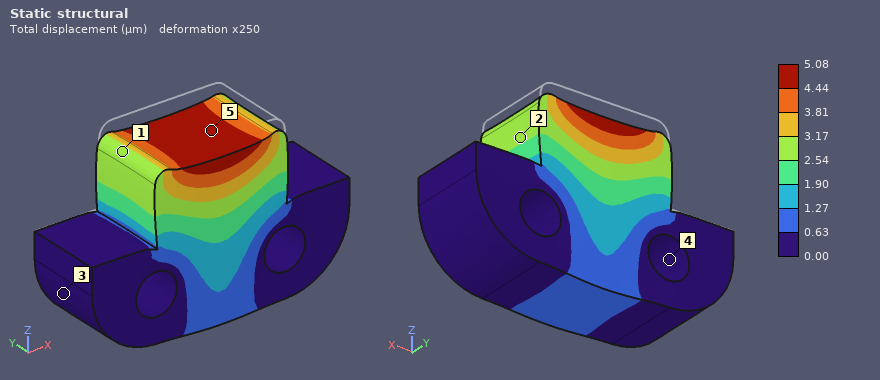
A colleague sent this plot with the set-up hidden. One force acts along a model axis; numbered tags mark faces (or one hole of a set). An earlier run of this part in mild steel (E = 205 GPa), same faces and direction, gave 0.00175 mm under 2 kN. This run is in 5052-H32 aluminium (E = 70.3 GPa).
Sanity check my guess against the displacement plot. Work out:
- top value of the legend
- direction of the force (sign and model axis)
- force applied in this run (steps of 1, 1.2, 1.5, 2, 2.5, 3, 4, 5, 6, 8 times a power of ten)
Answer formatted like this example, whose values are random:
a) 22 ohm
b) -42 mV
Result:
a) 5.08 µm
b) -Z
c) 2 kN
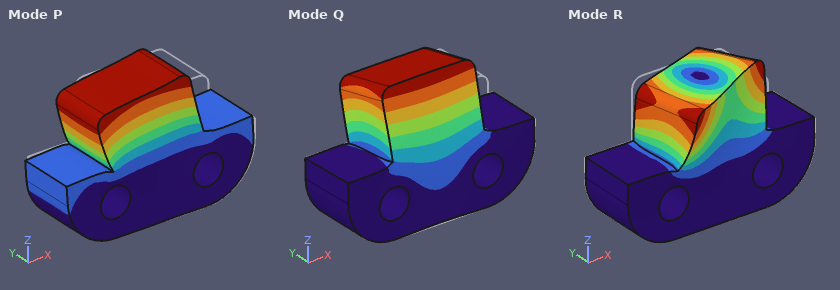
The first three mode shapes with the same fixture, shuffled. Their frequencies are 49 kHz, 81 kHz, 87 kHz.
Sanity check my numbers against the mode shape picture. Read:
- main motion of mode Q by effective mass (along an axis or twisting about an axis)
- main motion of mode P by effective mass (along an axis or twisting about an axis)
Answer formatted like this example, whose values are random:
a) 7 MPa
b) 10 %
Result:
a) along Y
b) along X
